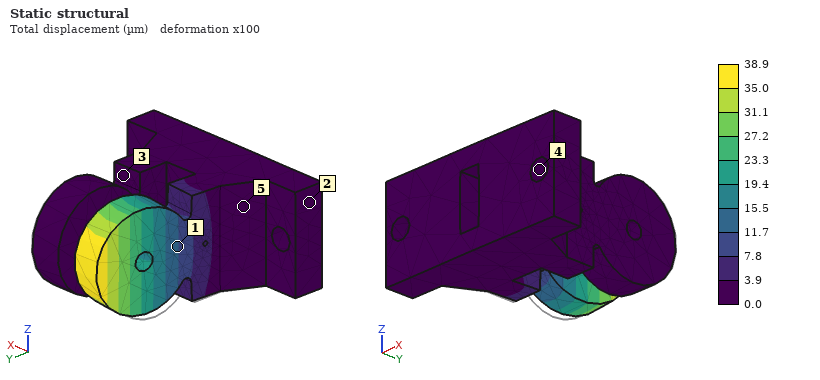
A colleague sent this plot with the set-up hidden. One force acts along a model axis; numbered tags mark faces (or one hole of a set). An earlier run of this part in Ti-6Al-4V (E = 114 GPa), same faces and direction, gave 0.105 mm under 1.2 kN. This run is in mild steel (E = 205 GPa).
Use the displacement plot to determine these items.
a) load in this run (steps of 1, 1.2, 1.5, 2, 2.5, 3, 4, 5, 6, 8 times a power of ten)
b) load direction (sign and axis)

800 N
+X
